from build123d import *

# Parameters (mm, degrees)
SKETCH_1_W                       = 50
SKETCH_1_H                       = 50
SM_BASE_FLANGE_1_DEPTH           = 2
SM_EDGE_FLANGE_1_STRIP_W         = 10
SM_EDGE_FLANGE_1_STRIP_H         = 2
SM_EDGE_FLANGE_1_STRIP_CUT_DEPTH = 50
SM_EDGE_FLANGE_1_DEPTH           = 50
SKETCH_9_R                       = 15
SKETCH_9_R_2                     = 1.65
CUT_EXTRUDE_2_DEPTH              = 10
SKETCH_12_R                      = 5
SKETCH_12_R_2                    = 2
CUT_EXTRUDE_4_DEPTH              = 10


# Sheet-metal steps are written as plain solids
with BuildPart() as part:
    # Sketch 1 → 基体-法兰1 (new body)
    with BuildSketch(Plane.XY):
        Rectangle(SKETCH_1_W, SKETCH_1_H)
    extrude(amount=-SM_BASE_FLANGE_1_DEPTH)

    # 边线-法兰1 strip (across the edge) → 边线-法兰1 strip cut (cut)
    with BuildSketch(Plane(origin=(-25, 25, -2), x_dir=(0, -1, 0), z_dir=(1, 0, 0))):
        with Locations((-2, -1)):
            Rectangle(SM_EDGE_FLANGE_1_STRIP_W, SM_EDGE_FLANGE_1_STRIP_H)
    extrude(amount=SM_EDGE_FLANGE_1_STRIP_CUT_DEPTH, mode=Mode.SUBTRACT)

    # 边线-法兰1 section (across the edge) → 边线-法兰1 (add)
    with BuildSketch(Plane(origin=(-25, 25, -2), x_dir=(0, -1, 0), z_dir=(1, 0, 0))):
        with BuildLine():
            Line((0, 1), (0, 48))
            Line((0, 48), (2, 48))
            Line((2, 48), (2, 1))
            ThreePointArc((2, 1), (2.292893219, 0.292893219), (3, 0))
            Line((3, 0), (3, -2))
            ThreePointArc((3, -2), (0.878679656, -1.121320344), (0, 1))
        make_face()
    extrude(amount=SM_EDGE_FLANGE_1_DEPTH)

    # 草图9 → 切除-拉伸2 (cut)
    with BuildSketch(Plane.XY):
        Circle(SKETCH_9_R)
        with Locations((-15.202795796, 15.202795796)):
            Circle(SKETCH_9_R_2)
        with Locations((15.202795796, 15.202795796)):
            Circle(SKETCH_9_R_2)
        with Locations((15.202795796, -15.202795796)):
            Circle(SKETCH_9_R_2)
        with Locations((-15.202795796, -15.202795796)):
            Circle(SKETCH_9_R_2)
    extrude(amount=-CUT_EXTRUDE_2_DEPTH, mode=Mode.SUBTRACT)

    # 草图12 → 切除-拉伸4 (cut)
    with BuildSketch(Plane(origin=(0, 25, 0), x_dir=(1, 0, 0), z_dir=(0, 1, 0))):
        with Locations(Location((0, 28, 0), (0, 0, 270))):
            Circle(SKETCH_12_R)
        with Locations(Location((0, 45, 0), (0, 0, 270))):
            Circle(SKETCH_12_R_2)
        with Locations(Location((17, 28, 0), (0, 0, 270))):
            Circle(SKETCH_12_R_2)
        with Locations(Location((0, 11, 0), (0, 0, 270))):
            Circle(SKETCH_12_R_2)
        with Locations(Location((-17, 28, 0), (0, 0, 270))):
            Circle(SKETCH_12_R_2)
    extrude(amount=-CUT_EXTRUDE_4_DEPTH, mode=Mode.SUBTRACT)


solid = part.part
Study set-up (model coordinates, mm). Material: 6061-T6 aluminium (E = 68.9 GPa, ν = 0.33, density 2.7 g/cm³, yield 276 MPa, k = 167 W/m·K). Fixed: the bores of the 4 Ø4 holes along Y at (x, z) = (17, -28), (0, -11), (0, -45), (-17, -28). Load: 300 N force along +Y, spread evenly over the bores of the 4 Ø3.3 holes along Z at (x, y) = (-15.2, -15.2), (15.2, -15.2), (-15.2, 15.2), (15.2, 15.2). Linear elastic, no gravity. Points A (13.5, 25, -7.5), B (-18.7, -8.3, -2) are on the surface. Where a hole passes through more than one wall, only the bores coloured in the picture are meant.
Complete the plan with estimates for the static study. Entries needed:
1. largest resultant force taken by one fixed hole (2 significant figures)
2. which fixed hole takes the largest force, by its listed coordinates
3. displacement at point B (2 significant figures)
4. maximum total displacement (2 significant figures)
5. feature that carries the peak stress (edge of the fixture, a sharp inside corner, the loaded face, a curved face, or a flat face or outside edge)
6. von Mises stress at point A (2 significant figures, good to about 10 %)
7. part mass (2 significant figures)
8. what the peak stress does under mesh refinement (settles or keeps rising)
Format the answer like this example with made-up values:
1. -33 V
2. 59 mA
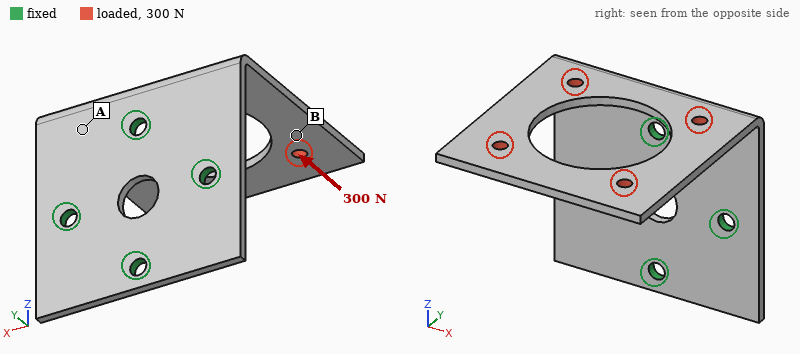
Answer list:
1. 350 N
2. (0, -11)
3. 0.25 mm
4. 0.38 mm
5. edge of the fixture
6. 29 MPa
7. 22 g
8. keeps rising
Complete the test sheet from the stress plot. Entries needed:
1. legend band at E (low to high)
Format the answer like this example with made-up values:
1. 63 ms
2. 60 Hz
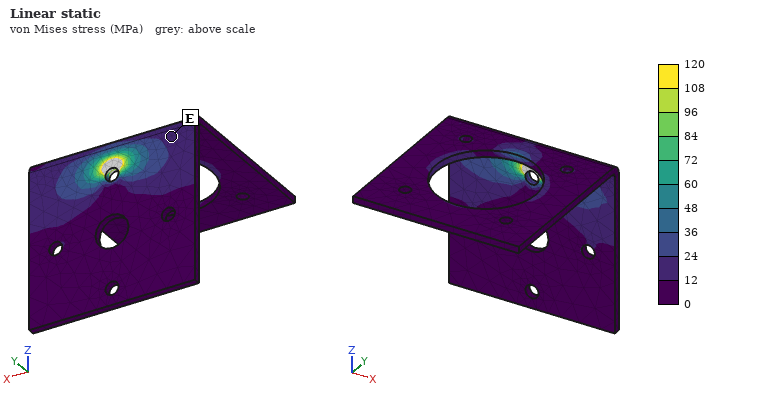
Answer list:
1. 12 to 24 MPa
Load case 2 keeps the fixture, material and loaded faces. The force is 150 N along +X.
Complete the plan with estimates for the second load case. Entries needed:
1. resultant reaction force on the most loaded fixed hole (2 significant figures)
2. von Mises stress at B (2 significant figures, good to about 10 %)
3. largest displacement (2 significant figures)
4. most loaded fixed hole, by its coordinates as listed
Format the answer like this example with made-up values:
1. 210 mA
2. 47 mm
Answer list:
1. 130 N
2. 11 MPa
3. 0.50 mm
4. (0, -11)
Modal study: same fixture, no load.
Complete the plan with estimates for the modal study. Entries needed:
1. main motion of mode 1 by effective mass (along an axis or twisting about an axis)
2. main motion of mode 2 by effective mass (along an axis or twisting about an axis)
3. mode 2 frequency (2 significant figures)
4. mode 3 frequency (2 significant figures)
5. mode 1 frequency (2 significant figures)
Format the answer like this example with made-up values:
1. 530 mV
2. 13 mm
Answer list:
1. along Z
2. along X
3. 930 Hz
4. 1300 Hz
5. 490 Hz
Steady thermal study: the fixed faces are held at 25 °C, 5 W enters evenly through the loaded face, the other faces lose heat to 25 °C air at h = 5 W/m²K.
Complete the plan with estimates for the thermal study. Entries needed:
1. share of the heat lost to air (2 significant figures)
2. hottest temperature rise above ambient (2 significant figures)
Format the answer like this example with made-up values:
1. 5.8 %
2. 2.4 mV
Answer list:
1. 5.4 %
2. 18 K
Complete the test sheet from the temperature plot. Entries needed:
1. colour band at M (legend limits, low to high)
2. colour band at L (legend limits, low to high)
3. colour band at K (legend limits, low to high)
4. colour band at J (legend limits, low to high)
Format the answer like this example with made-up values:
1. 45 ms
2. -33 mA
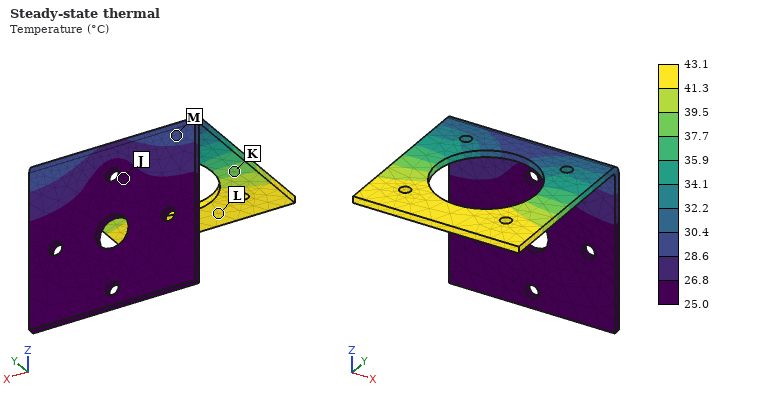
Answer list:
1. 28.6 to 30.4 °C
2. 41.3 to 43.1 °C
3. 37.7 to 39.5 °C
4. 25.0 to 26.8 °C
